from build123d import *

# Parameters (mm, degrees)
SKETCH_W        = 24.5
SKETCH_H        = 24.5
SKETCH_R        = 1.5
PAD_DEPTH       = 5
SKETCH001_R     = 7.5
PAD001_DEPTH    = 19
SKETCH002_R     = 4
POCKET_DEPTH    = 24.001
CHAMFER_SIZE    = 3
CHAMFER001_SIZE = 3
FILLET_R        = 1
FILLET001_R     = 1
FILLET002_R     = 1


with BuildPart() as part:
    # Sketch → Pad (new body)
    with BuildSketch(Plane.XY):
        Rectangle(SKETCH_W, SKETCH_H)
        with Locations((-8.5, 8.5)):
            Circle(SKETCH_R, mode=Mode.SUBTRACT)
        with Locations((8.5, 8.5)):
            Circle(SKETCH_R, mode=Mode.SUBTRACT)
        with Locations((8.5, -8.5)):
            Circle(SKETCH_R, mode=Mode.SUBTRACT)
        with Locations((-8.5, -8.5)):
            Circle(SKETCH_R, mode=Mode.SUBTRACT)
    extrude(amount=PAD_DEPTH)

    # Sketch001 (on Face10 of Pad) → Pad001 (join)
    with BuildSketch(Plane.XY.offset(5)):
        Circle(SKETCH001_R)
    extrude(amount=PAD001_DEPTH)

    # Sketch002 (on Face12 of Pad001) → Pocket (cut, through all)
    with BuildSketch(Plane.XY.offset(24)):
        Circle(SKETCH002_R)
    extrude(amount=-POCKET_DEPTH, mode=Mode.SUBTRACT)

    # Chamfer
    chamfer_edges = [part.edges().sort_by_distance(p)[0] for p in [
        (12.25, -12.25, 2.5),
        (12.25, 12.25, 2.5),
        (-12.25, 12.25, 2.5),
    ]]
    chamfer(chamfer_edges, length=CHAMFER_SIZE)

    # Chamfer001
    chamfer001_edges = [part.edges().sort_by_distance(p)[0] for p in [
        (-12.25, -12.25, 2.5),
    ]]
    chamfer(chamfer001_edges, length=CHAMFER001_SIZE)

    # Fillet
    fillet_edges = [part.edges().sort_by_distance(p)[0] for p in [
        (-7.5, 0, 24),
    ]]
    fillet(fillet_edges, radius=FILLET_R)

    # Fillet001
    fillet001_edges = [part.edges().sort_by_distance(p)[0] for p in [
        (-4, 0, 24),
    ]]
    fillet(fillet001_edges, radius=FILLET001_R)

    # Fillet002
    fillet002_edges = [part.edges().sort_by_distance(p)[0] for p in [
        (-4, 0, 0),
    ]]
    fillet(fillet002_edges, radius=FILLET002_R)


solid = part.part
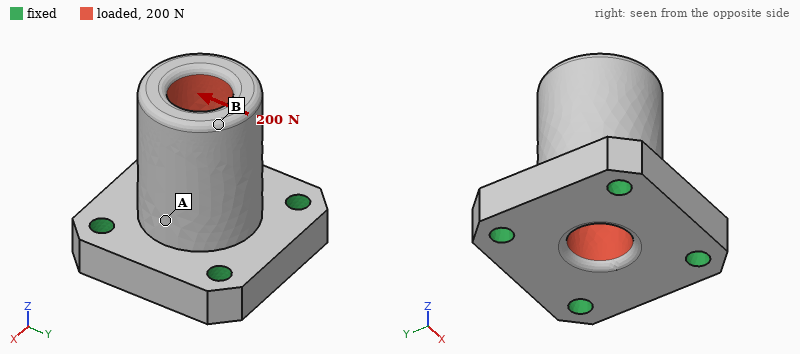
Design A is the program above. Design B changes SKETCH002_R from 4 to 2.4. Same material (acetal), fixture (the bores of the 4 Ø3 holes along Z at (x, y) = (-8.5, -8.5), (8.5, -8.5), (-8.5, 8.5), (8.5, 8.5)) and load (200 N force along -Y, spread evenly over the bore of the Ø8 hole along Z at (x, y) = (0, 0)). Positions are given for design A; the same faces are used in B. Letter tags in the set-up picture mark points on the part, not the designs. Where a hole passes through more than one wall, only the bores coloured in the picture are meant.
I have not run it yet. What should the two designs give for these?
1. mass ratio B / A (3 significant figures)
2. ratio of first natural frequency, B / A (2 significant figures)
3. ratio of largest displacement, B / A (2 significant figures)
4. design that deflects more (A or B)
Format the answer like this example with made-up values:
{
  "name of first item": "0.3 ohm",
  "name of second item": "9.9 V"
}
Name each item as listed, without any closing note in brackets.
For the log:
{
  "mass ratio B / A": "1.16",
  "ratio of first natural frequency, B / A": "0.96",
  "ratio of largest displacement, B / A": "0.89",
  "design that deflects more": "A"
}
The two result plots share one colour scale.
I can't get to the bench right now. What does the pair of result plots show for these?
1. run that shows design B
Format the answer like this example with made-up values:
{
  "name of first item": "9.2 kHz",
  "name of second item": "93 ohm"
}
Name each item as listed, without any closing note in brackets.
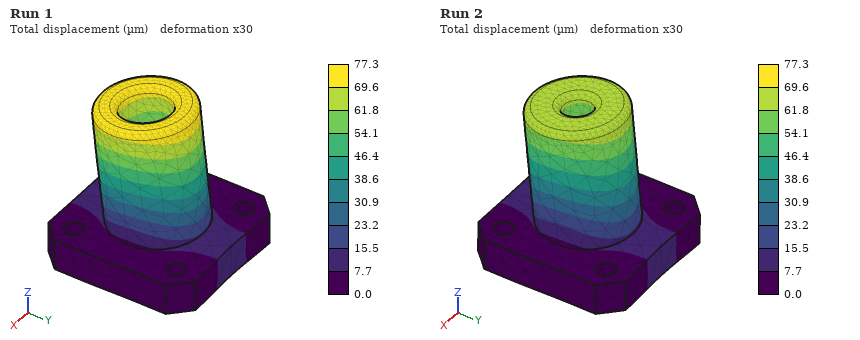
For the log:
{
  "run that shows design B": "Run 2"
}
